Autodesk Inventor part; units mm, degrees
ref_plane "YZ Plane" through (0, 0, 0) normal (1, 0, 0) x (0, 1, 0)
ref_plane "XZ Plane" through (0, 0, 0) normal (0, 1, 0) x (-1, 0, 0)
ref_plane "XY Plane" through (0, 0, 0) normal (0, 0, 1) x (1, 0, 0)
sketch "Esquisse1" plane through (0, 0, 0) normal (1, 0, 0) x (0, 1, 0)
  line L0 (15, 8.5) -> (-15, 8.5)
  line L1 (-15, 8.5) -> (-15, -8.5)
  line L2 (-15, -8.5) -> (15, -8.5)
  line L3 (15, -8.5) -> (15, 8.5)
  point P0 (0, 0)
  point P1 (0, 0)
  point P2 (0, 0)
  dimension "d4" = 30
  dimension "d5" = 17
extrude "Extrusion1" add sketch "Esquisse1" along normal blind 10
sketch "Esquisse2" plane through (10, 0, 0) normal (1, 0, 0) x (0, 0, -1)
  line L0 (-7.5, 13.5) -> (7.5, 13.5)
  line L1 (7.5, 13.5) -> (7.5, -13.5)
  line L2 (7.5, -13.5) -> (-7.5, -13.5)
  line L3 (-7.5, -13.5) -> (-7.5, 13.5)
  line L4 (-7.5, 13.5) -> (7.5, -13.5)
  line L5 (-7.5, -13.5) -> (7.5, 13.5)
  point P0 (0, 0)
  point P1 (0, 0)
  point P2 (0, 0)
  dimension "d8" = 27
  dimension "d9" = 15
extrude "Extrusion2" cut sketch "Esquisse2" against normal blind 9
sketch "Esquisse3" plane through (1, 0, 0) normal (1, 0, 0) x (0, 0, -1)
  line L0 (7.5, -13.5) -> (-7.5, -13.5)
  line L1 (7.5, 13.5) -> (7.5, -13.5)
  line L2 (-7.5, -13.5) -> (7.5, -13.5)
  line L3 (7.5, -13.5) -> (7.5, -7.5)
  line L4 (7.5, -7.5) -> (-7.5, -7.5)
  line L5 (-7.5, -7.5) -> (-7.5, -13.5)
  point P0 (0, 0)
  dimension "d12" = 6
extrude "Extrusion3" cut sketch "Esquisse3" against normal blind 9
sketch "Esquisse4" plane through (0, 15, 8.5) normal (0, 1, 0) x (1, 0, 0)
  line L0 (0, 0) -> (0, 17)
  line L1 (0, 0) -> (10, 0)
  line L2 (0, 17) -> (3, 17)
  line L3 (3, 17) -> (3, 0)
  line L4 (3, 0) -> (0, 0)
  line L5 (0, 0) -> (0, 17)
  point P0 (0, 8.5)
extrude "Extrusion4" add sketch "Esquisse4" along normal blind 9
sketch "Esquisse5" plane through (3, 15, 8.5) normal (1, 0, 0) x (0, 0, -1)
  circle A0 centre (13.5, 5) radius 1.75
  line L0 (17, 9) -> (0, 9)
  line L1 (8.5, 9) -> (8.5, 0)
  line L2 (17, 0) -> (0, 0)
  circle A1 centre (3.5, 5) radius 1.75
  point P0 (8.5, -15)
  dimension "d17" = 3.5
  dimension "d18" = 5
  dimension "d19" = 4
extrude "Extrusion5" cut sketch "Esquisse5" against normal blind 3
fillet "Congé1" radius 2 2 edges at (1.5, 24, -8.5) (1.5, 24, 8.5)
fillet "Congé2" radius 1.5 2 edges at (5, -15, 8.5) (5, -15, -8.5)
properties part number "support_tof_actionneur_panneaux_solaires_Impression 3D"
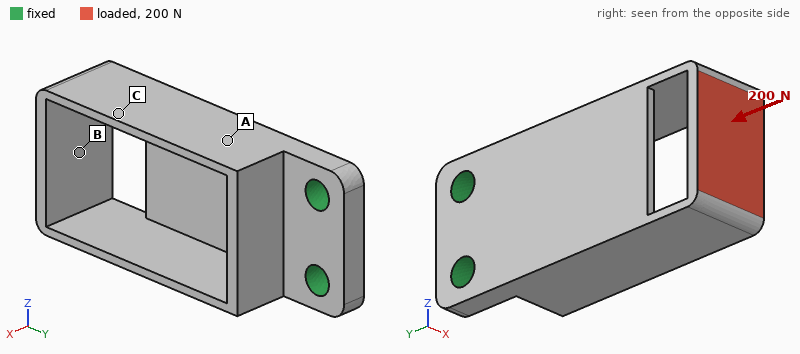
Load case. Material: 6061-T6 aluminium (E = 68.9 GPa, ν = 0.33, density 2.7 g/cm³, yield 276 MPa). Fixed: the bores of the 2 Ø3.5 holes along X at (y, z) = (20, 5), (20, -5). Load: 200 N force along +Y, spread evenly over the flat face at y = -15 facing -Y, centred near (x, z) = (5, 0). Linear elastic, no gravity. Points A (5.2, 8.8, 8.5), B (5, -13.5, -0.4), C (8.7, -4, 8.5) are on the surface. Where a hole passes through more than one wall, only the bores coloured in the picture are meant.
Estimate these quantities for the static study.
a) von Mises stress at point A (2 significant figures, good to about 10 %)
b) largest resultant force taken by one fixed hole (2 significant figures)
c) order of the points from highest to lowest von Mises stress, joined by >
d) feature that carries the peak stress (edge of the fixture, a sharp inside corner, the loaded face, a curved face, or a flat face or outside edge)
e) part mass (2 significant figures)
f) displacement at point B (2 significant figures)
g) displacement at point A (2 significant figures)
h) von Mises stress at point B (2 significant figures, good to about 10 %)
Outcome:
16 MPa
100 N
B > A > C
a flat face or outside edge
4.7 g
0.094 mm
0.021 mm
75 MPa
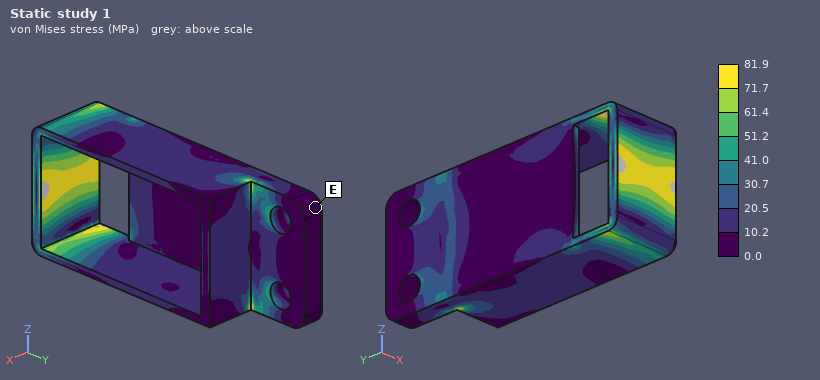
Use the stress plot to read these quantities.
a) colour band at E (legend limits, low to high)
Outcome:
0.0 to 10.2 MPa
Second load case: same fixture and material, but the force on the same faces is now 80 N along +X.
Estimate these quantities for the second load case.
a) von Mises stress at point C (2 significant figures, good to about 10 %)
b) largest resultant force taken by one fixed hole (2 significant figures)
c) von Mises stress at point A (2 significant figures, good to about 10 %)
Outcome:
18 MPa
79 N
24 MPa
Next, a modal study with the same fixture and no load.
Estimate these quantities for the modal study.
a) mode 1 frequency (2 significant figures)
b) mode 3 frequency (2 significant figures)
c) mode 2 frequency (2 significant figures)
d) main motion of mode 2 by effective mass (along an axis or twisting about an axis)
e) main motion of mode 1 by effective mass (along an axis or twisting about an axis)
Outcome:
2300 Hz
6300 Hz
3000 Hz
along Z
along X
